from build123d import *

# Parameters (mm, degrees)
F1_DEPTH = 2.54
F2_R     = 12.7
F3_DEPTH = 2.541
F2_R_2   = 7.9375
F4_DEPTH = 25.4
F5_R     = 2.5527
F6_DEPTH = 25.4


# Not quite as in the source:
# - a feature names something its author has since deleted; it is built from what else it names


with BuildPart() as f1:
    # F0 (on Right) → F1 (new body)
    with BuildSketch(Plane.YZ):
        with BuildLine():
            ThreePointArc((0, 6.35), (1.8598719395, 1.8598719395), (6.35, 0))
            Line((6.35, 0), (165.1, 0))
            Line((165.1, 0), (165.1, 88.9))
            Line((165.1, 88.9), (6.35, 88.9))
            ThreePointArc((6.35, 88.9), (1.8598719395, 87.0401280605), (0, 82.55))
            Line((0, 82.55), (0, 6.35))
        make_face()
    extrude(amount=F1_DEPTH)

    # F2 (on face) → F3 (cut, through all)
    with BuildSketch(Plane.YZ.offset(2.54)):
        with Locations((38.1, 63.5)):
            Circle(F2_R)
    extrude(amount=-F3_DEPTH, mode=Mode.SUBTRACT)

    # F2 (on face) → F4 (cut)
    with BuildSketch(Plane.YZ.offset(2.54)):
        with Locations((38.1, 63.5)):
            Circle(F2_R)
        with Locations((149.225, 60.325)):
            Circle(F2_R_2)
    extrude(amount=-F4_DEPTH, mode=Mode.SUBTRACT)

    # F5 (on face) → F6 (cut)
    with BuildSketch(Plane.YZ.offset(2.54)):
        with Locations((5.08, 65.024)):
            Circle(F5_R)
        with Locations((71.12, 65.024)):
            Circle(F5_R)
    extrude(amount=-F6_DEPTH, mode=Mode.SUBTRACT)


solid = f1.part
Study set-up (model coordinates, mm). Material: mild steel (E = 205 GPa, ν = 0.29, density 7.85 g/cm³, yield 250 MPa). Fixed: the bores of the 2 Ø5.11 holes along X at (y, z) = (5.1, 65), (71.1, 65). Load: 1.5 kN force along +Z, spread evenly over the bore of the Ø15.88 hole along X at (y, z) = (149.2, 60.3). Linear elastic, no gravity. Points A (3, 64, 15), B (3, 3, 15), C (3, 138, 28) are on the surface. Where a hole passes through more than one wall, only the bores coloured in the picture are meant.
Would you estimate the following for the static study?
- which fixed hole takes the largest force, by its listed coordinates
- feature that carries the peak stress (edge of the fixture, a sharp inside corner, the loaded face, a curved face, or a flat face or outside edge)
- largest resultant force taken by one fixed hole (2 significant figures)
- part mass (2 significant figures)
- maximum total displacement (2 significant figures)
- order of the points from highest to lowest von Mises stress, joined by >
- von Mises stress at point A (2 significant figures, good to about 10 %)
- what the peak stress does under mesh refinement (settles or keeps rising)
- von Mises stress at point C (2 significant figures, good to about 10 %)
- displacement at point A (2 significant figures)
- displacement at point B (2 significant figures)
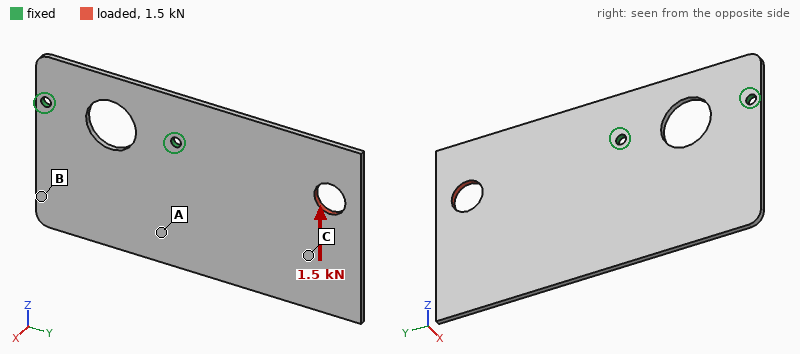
(71.1, 65)
edge of the fixture
3.2 kN
280 g
56 µm
A > C > B
21 MPa
keeps rising
13 MPa
15 µm
12 µm
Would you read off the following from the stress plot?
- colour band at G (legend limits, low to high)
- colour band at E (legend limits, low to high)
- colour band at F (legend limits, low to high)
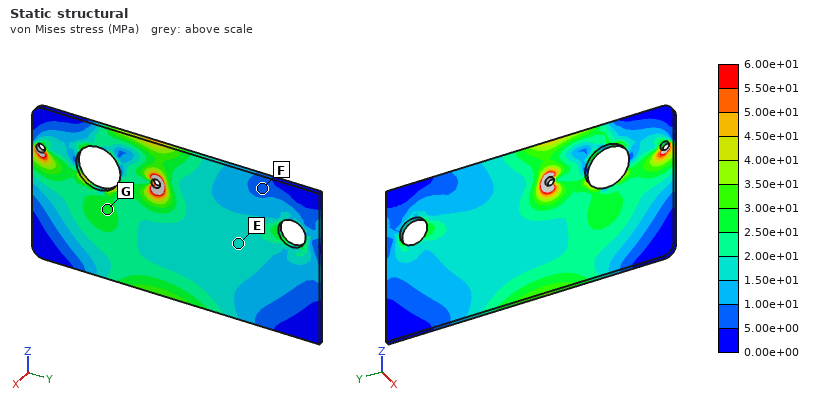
2.50e+01 to 3.00e+01 MPa
1.50e+01 to 2.00e+01 MPa
5.00e+00 to 1.00e+01 MPa
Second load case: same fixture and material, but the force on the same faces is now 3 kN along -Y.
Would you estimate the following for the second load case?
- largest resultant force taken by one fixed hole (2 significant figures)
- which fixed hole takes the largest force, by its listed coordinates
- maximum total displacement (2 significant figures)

2.5 kN
(71.1, 65)
15 µm
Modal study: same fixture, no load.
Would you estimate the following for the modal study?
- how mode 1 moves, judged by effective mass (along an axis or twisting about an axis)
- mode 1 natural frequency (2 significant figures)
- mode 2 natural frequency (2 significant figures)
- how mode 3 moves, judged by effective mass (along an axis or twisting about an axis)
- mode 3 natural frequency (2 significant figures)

along X
200 Hz
370 Hz
along X
610 Hz
